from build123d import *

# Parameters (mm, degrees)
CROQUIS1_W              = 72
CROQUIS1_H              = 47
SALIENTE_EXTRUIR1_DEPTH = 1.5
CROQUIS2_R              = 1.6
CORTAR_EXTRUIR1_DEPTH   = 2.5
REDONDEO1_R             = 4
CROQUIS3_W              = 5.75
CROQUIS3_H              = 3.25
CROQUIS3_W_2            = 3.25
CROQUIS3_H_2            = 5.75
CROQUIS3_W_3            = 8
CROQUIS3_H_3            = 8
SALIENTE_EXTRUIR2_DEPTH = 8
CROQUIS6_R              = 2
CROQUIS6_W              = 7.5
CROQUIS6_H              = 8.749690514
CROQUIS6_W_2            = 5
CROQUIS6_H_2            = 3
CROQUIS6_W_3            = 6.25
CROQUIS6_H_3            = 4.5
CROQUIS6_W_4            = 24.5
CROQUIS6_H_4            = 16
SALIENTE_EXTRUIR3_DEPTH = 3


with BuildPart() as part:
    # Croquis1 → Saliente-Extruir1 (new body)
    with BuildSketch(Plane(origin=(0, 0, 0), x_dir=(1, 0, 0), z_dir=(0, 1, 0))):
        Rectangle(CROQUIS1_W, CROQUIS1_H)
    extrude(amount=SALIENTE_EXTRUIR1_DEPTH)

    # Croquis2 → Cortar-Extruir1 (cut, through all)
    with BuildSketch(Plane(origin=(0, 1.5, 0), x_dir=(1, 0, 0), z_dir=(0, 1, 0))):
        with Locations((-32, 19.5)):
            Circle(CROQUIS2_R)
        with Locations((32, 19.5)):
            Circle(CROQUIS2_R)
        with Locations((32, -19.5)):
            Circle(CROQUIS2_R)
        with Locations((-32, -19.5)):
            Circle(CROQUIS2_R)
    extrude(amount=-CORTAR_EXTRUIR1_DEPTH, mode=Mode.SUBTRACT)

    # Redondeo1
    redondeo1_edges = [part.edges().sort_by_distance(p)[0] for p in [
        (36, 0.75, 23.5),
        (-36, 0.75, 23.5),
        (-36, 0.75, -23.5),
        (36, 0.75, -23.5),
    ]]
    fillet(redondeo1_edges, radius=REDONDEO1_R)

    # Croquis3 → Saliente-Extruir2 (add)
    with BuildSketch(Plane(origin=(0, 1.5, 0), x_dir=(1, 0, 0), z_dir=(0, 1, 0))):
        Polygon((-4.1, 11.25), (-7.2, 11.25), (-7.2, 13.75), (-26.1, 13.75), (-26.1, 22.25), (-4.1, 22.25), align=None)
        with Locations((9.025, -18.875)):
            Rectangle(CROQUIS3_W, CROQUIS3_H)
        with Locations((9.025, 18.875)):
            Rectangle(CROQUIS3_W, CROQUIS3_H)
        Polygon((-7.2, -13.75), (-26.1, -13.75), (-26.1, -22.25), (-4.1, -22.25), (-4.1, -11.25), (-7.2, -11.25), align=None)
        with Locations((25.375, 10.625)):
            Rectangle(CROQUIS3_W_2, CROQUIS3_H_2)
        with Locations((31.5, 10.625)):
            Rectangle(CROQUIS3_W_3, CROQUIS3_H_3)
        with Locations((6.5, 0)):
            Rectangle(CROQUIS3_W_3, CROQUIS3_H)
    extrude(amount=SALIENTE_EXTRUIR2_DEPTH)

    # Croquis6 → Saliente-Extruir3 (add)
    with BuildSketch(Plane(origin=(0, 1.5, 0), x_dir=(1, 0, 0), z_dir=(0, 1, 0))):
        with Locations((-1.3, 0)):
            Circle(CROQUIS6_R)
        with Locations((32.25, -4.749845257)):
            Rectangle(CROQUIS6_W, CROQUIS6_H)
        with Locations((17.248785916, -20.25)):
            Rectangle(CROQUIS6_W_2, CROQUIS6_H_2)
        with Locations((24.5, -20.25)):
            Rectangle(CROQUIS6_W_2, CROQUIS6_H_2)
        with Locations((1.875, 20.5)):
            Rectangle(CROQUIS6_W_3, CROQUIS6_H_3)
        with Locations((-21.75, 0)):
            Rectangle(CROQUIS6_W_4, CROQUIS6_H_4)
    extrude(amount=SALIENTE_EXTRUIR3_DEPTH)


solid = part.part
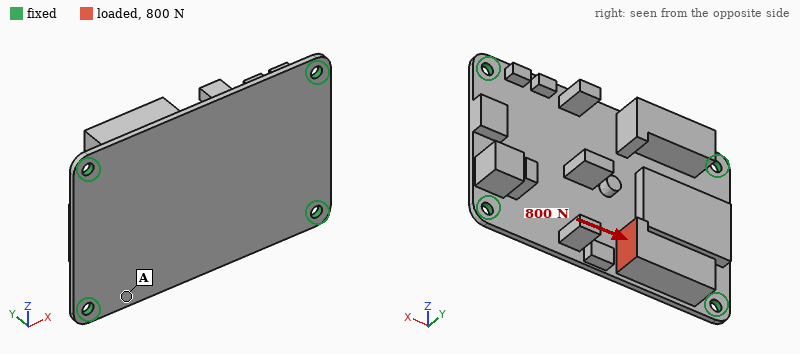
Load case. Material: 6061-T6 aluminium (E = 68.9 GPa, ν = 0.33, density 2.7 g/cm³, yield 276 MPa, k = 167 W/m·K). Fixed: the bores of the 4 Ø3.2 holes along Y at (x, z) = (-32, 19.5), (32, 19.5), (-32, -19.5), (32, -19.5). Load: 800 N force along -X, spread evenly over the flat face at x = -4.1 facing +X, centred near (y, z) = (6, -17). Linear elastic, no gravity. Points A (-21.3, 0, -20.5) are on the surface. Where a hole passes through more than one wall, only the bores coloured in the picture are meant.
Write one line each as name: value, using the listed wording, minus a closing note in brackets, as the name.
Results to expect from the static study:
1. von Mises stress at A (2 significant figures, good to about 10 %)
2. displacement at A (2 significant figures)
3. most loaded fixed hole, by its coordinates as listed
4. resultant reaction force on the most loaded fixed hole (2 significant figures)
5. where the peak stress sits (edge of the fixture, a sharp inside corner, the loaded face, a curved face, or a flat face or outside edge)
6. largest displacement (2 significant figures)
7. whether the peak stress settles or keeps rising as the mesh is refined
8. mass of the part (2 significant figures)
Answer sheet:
von Mises stress at A: 16 MPa
displacement at A: 0.062 mm
most loaded fixed hole, by its coordinates as listed: (-32, -19.5)
resultant reaction force on the most loaded fixed hole: 410 N
where the peak stress sits: edge of the fixture
largest displacement: 0.23 mm
whether the peak stress settles or keeps rising as the mesh is refined: keeps rising
mass of the part: 29 g
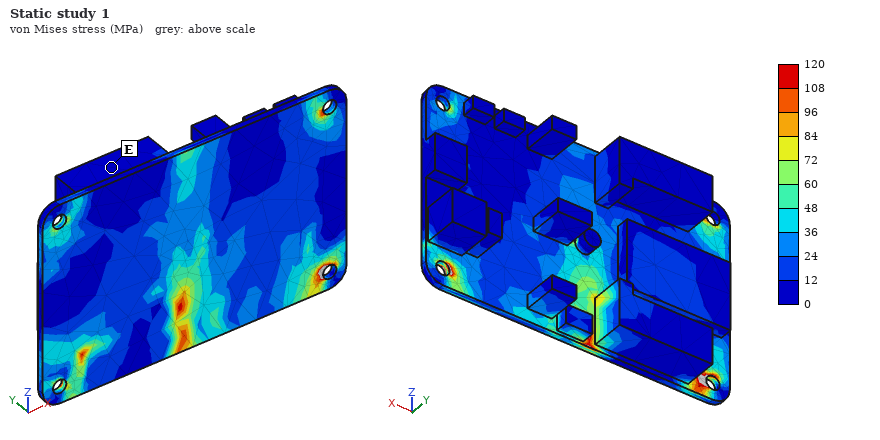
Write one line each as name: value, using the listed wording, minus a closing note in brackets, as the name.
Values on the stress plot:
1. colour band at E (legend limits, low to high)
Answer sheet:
colour band at E: 0 to 12 MPa
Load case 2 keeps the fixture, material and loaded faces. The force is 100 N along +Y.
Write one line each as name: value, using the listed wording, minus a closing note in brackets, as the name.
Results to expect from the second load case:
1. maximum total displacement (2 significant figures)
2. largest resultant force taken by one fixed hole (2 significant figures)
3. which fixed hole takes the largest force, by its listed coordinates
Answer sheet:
maximum total displacement: 0.15 mm
largest resultant force taken by one fixed hole: 77 N
which fixed hole takes the largest force, by its listed coordinates: (-32, -19.5)
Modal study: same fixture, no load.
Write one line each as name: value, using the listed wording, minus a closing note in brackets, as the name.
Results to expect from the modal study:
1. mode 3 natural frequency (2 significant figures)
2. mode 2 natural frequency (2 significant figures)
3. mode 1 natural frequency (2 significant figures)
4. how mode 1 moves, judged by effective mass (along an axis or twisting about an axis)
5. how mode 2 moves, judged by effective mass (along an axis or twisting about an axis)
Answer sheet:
mode 3 natural frequency: 3900 Hz
mode 2 natural frequency: 2900 Hz
mode 1 natural frequency: 1400 Hz
how mode 1 moves, judged by effective mass: along Y
how mode 2 moves, judged by effective mass: twisting about X
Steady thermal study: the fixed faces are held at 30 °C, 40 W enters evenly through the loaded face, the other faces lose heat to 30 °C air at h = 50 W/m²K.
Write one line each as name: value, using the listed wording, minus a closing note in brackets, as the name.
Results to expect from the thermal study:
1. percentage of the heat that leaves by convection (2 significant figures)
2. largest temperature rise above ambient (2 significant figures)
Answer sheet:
percentage of the heat that leaves by convection: 24 %
largest temperature rise above ambient: 74 K
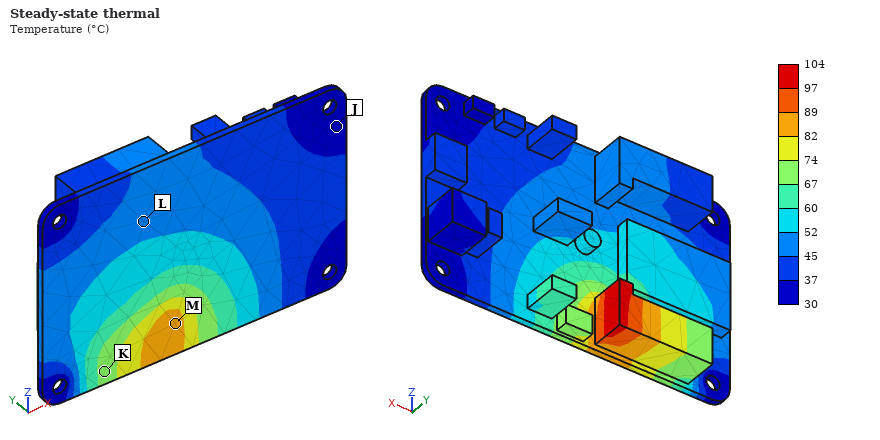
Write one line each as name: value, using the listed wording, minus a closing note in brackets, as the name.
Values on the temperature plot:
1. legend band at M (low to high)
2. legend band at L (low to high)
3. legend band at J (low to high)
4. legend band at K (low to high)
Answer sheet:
legend band at M: 82 to 89 °C
legend band at L: 45 to 52 °C
legend band at J: 30 to 37 °C
legend band at K: 67 to 74 °C
